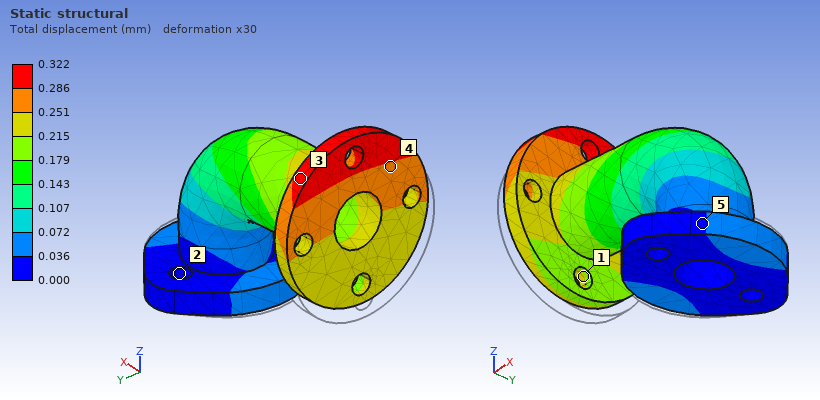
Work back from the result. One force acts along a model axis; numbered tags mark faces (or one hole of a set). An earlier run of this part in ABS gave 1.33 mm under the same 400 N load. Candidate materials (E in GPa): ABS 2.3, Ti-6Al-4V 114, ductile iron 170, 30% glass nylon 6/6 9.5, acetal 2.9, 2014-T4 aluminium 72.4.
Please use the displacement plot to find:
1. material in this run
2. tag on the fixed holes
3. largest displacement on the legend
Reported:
30% glass nylon 6/6
2
0.322 mm
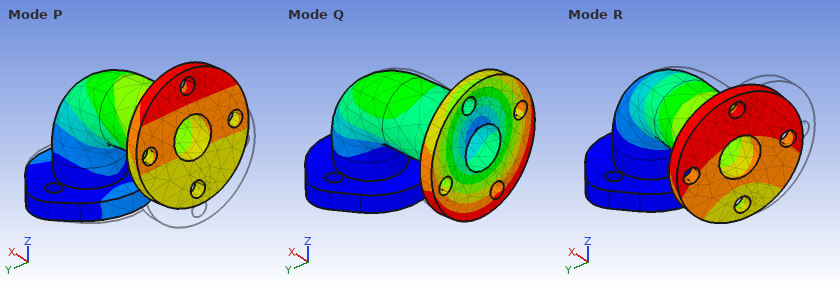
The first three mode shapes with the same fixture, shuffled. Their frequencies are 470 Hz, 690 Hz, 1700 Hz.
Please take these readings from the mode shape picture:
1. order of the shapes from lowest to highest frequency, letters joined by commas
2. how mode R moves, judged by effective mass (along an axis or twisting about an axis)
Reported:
P, R, Q
along Y
